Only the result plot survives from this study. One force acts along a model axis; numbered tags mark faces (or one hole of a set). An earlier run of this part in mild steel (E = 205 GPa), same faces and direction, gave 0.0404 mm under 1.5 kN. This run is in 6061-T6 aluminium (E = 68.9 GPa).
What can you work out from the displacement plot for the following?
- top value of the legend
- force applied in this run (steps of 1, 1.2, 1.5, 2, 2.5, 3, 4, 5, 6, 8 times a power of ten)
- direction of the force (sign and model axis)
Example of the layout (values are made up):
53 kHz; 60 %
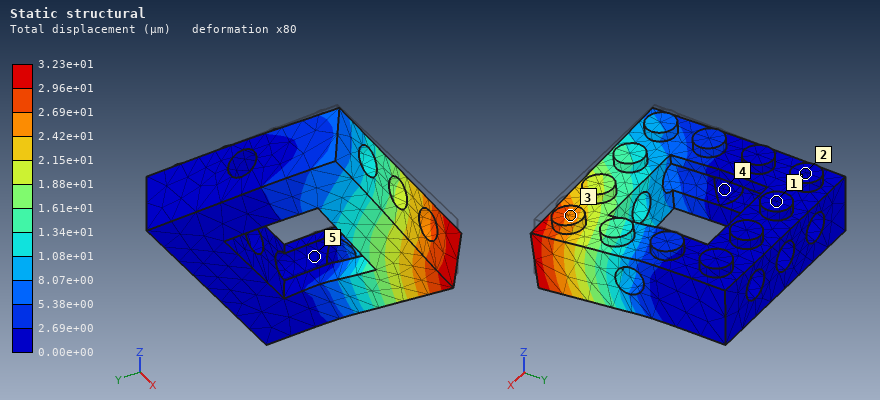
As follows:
3.23e+01 µm; 400 N; -Z
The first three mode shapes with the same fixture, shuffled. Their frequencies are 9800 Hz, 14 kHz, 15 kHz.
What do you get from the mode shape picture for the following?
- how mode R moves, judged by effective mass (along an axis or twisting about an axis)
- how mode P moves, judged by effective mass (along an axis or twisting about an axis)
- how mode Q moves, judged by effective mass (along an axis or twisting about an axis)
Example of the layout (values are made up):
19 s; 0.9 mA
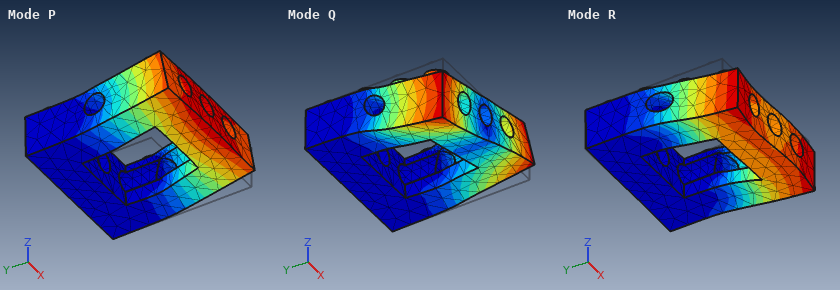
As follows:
along X; along Z; twisting about Y
